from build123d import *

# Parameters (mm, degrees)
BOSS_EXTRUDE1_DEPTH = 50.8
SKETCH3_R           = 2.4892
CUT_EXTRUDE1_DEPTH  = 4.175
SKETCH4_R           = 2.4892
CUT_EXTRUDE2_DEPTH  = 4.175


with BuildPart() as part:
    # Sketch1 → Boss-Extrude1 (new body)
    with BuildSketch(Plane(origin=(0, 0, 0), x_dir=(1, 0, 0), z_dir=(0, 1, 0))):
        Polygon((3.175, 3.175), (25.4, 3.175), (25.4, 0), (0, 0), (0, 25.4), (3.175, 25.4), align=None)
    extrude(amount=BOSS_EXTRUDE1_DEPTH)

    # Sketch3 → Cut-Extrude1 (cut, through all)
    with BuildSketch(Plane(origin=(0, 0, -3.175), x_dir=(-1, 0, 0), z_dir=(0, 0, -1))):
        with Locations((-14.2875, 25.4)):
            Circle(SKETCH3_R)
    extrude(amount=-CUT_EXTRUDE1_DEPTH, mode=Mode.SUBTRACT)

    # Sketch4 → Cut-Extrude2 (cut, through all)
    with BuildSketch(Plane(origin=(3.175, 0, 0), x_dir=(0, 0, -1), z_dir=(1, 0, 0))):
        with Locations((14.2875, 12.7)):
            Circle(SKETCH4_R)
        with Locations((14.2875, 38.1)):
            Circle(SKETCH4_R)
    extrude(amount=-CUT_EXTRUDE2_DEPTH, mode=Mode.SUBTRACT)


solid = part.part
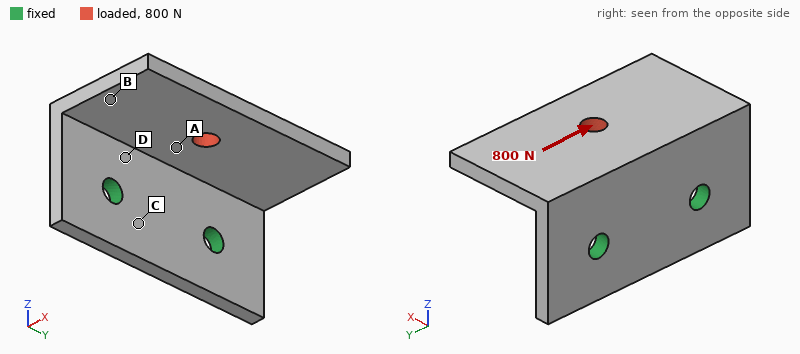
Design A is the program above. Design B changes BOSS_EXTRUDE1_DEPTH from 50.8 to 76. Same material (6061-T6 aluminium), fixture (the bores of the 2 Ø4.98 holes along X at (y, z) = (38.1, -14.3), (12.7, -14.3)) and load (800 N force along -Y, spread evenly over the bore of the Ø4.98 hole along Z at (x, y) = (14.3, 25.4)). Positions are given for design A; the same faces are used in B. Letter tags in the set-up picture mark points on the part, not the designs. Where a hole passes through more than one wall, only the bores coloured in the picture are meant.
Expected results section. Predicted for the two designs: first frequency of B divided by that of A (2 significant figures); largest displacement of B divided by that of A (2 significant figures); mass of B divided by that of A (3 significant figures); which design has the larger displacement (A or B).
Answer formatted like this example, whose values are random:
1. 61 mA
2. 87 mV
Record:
1. 0.81
2. 1.4
3. 1.51
4. B
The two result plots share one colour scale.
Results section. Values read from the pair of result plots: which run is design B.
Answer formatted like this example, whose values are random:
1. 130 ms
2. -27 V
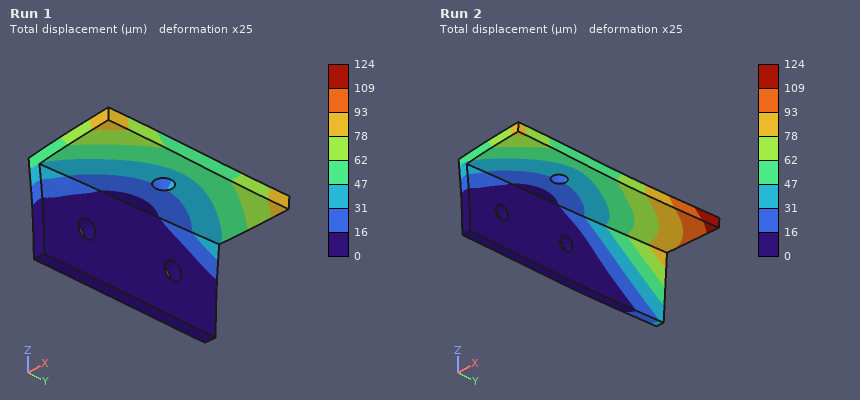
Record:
1. Run 2
